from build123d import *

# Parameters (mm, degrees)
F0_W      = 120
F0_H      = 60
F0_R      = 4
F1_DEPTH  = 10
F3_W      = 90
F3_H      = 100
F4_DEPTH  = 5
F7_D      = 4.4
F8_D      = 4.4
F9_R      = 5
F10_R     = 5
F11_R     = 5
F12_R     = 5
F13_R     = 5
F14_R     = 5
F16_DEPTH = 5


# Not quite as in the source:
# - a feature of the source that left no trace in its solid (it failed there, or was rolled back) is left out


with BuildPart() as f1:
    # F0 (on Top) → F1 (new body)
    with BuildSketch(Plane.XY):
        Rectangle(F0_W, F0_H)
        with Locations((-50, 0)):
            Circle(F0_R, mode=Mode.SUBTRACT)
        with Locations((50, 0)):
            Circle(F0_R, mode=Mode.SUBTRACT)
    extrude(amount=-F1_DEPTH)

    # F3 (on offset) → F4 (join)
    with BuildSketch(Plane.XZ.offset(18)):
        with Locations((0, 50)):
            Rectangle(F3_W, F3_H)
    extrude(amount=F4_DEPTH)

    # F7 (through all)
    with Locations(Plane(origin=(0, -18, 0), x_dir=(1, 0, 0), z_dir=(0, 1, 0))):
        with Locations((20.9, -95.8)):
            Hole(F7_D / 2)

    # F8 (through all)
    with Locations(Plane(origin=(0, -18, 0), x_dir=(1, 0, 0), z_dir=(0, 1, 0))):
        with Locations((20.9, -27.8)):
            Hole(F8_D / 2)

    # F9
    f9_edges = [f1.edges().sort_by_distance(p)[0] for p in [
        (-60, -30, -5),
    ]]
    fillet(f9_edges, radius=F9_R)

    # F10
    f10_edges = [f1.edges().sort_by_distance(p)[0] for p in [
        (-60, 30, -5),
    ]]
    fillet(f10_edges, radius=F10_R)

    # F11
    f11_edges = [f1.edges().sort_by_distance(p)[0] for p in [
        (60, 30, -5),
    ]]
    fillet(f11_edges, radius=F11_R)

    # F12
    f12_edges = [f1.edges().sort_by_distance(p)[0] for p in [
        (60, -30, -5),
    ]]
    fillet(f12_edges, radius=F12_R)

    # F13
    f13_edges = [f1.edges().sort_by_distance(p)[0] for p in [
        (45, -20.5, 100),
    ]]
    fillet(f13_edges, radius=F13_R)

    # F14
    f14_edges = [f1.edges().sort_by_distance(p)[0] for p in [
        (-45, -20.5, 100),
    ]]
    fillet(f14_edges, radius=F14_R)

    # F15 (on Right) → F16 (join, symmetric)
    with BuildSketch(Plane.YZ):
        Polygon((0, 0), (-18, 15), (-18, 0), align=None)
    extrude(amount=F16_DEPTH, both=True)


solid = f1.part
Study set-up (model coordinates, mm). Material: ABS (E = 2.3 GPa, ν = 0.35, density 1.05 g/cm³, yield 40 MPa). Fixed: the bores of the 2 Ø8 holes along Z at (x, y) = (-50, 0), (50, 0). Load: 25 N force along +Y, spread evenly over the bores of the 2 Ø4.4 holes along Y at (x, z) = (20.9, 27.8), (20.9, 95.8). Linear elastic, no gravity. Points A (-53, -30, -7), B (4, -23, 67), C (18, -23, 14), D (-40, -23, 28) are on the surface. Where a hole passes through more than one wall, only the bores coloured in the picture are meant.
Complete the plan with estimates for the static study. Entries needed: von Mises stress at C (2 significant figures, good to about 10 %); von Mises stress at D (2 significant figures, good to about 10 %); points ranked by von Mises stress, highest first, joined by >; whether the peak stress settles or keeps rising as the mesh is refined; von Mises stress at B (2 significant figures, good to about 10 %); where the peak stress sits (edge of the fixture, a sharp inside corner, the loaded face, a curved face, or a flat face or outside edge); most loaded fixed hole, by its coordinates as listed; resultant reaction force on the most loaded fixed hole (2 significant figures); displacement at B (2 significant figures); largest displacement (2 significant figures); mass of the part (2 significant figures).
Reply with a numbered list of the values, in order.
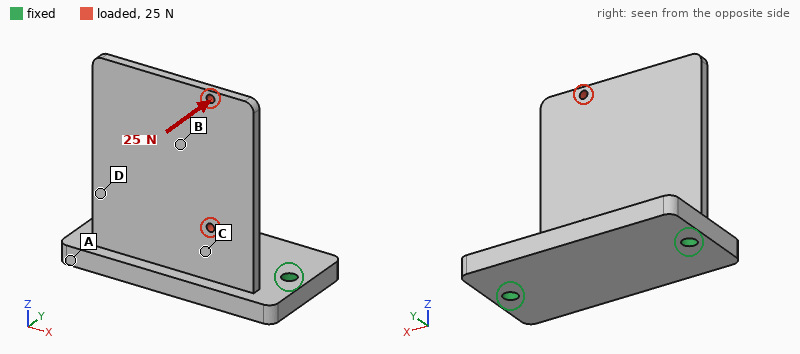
1. 2.9 MPa
2. 2.2 MPa
3. C > D > B > A
4. keeps rising
5. 1.1 MPa
6. a sharp inside corner
7. (50, 0)
8. 18 N
9. 0.99 mm
10. 2.1 mm
11. 120 g
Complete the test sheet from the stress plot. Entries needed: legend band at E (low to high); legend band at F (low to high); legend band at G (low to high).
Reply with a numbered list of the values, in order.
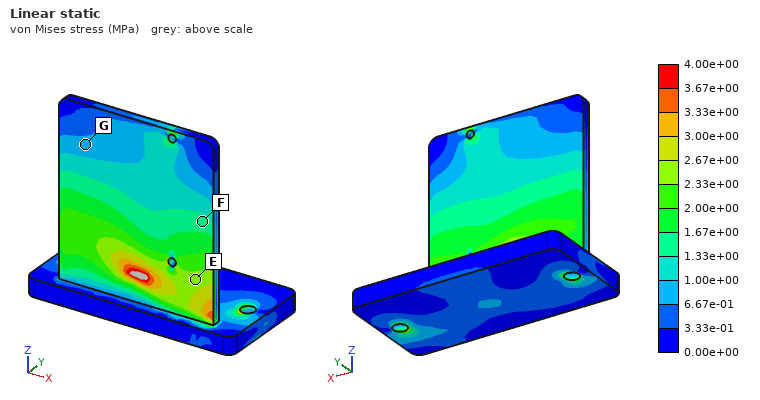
1. 2.33e+00 to 2.67e+00 MPa
2. 1.33e+00 to 1.67e+00 MPa
3. 6.67e-01 to 1.00e+00 MPa
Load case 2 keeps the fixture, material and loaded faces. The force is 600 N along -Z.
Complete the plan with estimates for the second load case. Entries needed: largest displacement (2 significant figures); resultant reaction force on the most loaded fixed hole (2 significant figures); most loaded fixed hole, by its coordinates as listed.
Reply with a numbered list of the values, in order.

1. 1.1 mm
2. 440 N
3. (50, 0)
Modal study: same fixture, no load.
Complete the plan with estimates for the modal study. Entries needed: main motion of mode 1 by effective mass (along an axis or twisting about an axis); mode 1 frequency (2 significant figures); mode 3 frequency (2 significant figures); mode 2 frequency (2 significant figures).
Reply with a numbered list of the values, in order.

1. along Y
2. 130 Hz
3. 690 Hz
4. 310 Hz
